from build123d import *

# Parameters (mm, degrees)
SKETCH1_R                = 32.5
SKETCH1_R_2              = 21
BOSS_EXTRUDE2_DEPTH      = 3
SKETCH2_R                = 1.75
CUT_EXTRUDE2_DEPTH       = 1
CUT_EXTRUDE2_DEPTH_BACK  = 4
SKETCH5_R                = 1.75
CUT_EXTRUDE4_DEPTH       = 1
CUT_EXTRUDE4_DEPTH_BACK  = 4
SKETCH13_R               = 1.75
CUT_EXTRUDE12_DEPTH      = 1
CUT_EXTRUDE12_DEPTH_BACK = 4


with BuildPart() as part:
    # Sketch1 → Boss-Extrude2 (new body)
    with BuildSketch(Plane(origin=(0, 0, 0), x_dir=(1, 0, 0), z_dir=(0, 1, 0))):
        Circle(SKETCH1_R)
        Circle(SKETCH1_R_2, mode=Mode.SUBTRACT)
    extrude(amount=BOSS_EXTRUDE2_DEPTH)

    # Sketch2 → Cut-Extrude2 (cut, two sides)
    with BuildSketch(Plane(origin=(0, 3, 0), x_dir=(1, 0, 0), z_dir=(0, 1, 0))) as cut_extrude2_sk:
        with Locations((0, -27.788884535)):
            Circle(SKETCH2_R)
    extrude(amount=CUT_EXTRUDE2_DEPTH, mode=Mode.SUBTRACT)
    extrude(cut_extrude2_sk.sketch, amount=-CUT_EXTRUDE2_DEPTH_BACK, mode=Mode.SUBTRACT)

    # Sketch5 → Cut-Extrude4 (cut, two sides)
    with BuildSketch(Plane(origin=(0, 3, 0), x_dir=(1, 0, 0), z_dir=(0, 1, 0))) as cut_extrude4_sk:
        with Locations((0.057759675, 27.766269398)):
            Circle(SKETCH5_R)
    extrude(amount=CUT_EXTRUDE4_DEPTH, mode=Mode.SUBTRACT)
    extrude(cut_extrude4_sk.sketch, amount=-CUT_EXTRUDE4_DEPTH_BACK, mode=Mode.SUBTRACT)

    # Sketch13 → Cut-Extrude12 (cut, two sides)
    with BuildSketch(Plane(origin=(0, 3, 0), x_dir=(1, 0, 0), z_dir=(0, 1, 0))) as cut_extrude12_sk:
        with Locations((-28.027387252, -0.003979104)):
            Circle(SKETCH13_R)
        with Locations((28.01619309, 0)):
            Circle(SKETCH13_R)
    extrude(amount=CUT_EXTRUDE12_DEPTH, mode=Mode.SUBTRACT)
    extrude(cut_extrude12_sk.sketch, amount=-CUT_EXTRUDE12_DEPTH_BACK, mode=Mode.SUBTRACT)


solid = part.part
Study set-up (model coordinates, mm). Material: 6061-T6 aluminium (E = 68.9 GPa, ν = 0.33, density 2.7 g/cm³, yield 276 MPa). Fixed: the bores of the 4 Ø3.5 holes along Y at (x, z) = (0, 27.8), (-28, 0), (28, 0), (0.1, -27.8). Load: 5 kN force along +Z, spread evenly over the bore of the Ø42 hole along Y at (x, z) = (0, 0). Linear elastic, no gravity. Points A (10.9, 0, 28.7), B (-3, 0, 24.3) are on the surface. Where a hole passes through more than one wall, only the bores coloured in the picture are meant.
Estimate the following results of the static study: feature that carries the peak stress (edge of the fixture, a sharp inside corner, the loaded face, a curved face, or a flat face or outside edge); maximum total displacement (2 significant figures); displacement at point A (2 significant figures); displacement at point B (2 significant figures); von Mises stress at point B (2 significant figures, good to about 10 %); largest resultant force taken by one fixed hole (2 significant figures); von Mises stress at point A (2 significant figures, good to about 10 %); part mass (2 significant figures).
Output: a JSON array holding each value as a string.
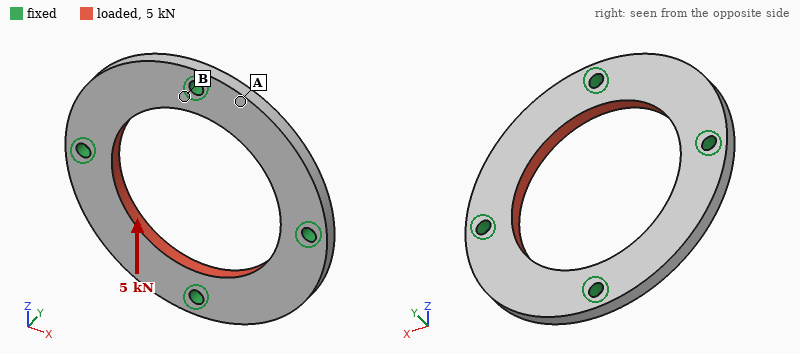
["edge of the fixture", "12 µm", "6.8 µm", "2.3 µm", "33 MPa", "1.6 kN", "12 MPa", "15 g"]
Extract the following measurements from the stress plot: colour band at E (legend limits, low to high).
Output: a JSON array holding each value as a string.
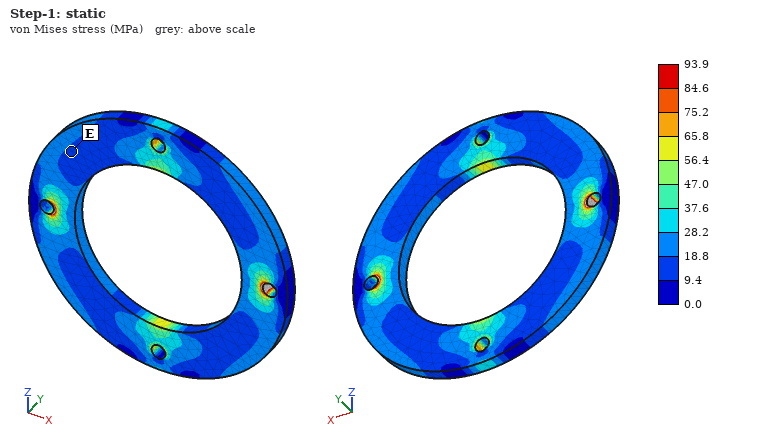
["9.4 to 18.8 MPa"]
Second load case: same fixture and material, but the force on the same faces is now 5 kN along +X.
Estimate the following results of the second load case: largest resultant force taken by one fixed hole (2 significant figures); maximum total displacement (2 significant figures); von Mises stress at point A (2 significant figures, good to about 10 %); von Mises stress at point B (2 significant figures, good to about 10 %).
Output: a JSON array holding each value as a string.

["1.6 kN", "11 µm", "19 MPa", "39 MPa"]
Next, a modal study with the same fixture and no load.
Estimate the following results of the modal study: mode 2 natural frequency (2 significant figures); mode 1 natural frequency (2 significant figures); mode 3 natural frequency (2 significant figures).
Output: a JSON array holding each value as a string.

["8100 Hz", "7800 Hz", "8100 Hz"]
